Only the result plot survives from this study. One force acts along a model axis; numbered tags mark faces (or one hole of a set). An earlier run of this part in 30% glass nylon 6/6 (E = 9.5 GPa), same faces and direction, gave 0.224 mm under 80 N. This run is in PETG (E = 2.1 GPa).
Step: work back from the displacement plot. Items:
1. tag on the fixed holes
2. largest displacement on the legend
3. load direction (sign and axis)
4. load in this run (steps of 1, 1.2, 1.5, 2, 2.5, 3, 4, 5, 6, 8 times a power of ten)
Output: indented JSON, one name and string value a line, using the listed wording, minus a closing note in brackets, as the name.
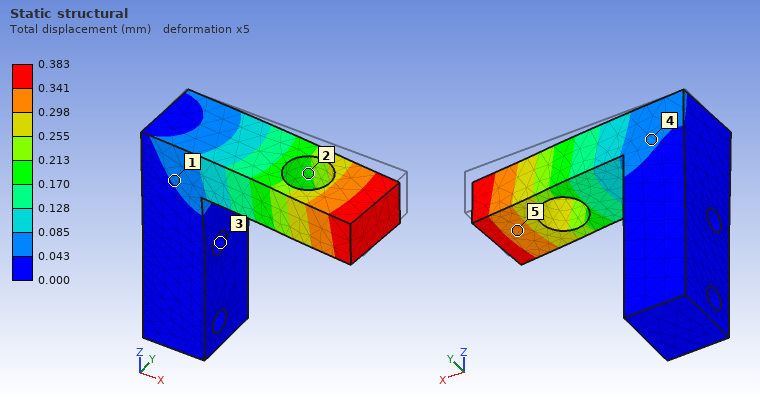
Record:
{
  "tag on the fixed holes": "3",
  "largest displacement on the legend": "0.383 mm",
  "load direction": "-Y",
  "load in this run": "30 N"
}
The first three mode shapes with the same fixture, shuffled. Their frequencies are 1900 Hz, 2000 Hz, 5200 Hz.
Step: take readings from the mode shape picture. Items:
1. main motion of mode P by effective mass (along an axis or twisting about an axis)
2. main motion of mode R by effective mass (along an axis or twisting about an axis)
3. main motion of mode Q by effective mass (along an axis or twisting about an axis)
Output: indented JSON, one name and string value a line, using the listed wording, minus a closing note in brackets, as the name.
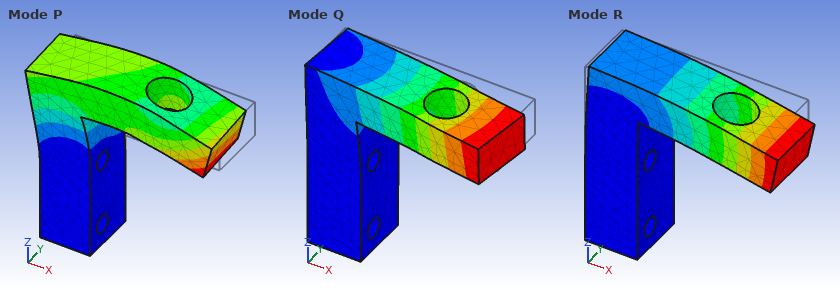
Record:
{
  "main motion of mode P by effective mass": "along X",
  "main motion of mode R by effective mass": "along Z",
  "main motion of mode Q by effective mass": "along Y"
}
